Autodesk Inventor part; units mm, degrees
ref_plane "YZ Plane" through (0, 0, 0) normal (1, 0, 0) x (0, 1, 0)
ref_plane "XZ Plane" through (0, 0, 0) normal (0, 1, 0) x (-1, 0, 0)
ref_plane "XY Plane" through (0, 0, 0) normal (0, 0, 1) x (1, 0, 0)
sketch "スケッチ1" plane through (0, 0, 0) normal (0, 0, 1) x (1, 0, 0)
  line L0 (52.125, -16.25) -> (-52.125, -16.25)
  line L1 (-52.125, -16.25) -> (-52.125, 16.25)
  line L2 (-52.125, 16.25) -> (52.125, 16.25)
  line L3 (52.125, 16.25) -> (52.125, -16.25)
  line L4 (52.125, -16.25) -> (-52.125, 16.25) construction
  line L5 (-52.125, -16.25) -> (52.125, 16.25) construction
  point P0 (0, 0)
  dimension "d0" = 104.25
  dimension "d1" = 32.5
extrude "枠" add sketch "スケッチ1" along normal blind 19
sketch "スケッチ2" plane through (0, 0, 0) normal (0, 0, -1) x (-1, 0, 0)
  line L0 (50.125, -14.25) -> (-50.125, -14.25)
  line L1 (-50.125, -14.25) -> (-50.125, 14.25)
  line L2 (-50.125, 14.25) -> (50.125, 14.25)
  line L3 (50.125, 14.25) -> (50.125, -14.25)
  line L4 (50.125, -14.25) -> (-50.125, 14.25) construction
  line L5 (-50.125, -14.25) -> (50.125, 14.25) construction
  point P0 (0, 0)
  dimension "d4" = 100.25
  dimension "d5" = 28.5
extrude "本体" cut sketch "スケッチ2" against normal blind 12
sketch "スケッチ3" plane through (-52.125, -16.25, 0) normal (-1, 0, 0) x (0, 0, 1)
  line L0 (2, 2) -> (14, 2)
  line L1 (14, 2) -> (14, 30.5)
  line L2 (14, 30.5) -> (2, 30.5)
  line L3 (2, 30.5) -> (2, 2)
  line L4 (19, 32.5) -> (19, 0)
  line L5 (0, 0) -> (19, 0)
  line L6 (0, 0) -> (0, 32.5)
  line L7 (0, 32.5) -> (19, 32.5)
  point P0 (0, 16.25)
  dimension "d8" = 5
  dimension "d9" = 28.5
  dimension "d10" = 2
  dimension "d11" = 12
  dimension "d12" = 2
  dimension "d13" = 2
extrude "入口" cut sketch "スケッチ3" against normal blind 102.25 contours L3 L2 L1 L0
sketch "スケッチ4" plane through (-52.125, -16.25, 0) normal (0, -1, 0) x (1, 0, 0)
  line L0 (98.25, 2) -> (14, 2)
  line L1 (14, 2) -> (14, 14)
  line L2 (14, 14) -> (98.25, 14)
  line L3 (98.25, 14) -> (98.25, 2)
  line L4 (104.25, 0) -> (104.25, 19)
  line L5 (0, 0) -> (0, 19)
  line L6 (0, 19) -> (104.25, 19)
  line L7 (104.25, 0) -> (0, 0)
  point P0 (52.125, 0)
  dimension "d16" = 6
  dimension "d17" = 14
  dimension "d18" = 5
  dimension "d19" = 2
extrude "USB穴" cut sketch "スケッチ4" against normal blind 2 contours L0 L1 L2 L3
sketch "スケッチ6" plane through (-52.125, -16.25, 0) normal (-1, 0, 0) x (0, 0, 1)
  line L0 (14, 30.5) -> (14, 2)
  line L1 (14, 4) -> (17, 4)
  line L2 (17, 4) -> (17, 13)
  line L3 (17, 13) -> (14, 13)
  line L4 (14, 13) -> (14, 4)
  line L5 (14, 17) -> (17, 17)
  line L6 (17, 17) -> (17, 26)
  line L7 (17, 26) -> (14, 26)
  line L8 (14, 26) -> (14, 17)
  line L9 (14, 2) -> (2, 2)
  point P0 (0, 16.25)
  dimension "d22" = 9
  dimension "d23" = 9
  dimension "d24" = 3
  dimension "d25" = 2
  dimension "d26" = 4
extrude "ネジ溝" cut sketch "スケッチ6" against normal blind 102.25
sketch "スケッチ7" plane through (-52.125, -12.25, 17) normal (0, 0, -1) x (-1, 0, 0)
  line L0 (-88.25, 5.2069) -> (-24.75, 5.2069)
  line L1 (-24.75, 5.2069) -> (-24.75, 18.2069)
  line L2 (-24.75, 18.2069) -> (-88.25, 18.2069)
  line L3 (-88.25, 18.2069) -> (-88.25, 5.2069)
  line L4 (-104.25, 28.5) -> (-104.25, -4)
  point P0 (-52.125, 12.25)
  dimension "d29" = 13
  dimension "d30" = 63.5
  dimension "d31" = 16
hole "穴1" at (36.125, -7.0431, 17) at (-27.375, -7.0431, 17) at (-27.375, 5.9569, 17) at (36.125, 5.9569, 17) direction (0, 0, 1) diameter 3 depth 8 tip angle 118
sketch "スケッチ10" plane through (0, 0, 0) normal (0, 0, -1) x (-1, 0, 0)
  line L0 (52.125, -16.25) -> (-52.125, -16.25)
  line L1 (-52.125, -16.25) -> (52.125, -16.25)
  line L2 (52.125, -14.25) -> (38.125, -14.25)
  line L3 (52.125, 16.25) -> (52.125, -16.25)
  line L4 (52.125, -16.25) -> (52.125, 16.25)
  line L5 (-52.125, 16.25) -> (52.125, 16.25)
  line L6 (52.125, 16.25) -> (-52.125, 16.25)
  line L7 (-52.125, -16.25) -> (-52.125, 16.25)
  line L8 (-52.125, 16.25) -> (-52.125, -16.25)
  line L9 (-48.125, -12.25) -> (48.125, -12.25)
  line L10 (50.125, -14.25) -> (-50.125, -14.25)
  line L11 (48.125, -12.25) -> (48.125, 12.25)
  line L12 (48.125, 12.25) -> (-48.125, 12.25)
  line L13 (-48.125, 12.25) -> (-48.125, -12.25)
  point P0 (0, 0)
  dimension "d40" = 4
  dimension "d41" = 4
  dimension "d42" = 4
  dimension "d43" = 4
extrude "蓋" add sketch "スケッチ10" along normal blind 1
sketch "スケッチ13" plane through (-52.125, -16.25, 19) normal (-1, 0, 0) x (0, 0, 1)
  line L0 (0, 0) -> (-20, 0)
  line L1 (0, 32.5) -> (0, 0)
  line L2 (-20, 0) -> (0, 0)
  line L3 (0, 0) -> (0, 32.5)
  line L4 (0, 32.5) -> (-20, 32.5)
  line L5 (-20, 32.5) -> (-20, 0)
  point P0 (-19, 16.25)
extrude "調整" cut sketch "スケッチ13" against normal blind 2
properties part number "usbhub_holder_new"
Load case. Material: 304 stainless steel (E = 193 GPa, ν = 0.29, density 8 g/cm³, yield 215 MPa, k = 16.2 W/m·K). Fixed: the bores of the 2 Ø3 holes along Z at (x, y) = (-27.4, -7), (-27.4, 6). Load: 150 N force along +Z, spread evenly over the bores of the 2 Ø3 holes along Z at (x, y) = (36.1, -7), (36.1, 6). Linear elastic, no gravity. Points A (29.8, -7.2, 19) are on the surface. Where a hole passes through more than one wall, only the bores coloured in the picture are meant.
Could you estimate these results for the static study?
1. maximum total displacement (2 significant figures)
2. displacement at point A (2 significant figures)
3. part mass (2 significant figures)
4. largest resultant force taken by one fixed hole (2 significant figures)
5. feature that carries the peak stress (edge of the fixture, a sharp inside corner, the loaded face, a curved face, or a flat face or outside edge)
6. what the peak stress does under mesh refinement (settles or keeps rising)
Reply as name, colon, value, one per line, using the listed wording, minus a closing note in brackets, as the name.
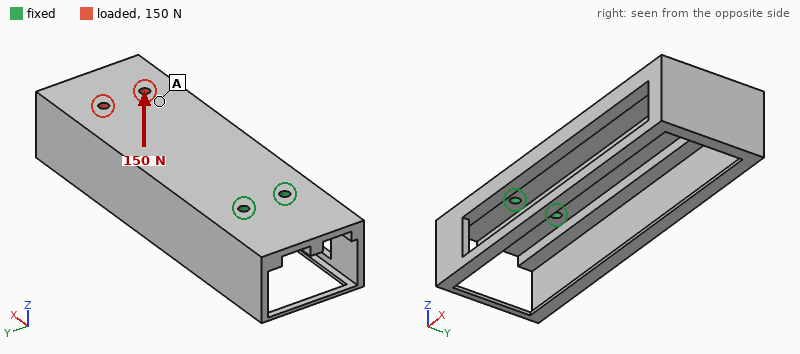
maximum total displacement: 0.40 mm
displacement at point A: 0.28 mm
part mass: 130 g
largest resultant force taken by one fixed hole: 83 N
feature that carries the peak stress: edge of the fixture
what the peak stress does under mesh refinement: keeps rising
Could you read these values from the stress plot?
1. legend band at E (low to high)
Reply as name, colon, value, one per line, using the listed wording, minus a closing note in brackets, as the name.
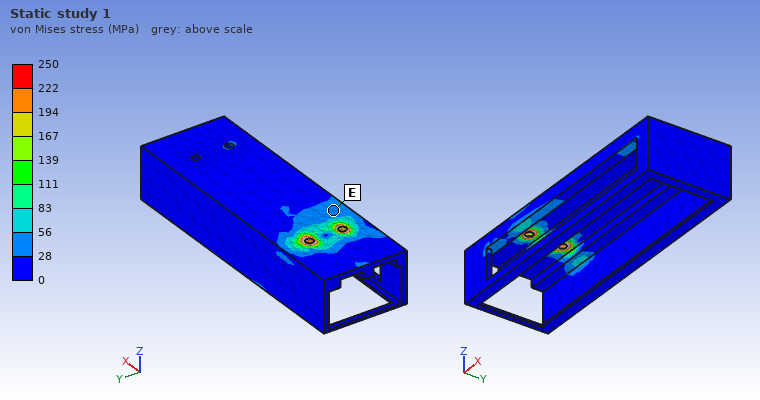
legend band at E: 28 to 56 MPa
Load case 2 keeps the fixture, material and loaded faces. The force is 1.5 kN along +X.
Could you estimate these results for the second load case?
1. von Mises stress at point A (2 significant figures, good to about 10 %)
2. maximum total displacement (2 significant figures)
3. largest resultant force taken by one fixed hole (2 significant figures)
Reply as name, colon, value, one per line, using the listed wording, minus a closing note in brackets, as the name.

von Mises stress at point A: 27 MPa
maximum total displacement: 31 µm
largest resultant force taken by one fixed hole: 750 N
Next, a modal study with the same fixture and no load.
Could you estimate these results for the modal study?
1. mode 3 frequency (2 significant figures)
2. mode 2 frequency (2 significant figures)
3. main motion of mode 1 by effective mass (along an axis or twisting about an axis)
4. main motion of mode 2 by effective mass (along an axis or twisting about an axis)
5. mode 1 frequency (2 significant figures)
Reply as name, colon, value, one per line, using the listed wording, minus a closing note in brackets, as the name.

mode 3 frequency: 1500 Hz
mode 2 frequency: 1000 Hz
main motion of mode 1 by effective mass: along Z
main motion of mode 2 by effective mass: along Y
mode 1 frequency: 440 Hz
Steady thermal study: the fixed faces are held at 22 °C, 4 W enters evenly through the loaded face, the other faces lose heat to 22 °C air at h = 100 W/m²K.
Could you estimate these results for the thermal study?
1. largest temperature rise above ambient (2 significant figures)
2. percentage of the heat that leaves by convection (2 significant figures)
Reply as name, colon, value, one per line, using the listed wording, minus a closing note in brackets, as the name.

largest temperature rise above ambient: 26 K
percentage of the heat that leaves by convection: 99 %
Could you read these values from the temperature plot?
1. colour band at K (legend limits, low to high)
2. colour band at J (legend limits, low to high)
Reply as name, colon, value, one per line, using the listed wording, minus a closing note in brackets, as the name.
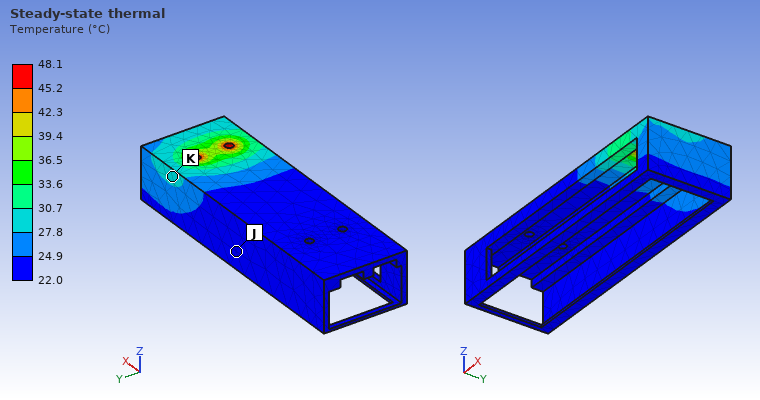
colour band at K: 27.8 to 30.7 °C
colour band at J: 22.0 to 24.9 °C
